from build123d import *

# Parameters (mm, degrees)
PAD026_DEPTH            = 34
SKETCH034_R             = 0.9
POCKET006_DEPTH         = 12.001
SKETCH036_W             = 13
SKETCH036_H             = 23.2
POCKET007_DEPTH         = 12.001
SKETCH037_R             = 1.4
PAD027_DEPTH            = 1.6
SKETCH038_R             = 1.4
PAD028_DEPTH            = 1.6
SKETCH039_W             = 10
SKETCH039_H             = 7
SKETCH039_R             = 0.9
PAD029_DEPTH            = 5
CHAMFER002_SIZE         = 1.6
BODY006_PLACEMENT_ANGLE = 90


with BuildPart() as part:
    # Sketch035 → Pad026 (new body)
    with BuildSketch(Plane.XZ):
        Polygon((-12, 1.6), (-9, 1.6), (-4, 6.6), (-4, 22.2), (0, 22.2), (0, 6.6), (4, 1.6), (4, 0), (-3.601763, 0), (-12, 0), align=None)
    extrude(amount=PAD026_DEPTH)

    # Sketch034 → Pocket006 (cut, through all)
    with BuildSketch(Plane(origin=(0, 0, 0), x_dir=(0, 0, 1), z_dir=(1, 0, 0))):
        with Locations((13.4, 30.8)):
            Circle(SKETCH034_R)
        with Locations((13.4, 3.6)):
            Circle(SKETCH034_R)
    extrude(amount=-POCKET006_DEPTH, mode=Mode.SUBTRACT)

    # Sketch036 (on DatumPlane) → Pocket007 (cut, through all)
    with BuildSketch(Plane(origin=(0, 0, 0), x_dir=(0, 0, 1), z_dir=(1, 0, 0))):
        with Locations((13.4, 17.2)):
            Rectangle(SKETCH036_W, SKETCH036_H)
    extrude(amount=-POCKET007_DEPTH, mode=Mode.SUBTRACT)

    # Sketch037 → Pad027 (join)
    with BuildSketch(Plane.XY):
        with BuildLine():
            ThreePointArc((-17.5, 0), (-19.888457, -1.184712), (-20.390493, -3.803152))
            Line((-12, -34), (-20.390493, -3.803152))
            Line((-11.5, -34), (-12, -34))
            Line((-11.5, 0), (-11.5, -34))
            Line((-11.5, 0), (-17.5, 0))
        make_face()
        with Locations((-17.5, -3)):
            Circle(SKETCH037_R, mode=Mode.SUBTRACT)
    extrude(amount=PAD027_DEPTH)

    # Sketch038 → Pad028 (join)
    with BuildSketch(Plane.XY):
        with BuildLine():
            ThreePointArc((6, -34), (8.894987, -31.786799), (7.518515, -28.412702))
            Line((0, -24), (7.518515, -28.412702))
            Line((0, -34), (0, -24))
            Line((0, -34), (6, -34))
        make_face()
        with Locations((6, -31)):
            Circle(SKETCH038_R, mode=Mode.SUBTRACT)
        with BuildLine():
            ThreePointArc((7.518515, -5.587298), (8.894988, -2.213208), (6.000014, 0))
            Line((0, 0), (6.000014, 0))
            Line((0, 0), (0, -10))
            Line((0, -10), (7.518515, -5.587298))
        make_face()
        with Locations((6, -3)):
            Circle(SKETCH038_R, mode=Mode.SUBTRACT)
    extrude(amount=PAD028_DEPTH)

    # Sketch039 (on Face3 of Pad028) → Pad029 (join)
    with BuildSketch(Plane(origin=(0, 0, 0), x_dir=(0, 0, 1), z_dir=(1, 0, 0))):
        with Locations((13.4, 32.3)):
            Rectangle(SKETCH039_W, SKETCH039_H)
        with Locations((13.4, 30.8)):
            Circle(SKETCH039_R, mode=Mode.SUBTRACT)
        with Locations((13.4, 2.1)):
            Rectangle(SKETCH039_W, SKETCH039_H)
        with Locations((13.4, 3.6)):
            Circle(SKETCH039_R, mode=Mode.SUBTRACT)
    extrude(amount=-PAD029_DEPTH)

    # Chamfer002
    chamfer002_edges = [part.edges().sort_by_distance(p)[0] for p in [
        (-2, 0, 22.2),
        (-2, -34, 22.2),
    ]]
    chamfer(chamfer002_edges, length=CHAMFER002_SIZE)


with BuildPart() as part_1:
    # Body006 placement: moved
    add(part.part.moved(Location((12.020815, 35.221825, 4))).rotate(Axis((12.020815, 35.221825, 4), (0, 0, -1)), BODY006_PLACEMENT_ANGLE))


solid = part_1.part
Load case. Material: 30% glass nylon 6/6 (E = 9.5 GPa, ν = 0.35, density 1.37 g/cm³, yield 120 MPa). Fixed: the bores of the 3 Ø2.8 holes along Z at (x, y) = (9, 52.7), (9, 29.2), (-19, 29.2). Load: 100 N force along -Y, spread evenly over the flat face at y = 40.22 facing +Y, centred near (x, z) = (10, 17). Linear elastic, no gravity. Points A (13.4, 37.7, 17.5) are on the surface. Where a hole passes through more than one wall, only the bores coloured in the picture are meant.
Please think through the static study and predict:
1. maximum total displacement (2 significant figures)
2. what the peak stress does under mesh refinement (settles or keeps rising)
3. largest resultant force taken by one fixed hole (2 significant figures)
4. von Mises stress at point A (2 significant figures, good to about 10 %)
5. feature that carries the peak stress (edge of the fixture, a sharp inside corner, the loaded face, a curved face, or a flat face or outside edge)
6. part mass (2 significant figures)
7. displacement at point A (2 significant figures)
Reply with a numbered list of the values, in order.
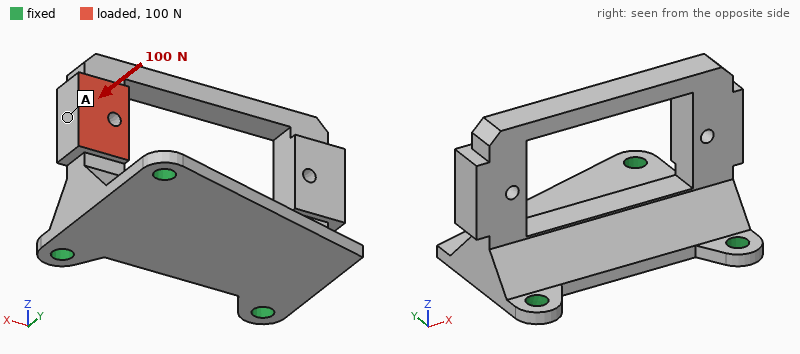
1. 0.31 mm
2. keeps rising
3. 81 N
4. 6.0 MPa
5. edge of the fixture
6. 5.2 g
7. 0.17 mm
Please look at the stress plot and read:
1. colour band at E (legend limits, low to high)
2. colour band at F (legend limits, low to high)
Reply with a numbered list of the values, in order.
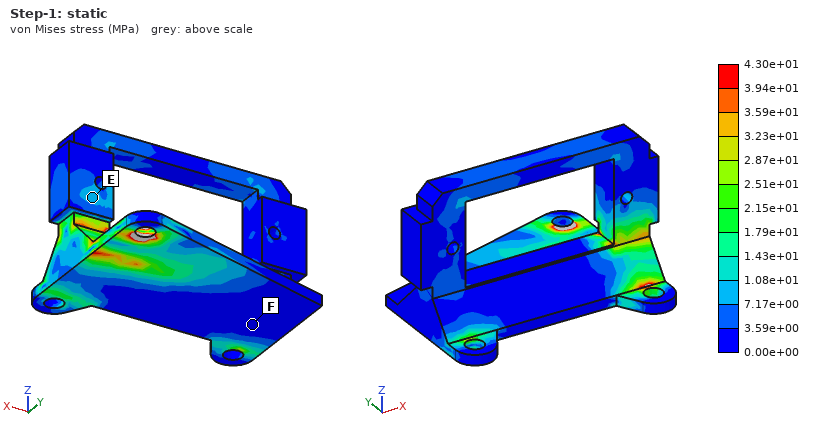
1. 7.17e+00 to 1.08e+01 MPa
2. 0.00e+00 to 3.59e+00 MPa
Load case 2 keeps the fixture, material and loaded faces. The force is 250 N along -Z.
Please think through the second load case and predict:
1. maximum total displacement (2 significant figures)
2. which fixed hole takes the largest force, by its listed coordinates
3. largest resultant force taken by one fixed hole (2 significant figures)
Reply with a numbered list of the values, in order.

1. 0.47 mm
2. (9, 29.2)
3. 170 N
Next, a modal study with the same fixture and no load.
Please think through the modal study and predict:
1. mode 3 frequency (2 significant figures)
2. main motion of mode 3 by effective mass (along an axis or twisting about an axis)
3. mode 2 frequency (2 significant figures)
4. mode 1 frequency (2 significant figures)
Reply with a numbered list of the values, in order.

1. 5100 Hz
2. along X
3. 3900 Hz
4. 2100 Hz
